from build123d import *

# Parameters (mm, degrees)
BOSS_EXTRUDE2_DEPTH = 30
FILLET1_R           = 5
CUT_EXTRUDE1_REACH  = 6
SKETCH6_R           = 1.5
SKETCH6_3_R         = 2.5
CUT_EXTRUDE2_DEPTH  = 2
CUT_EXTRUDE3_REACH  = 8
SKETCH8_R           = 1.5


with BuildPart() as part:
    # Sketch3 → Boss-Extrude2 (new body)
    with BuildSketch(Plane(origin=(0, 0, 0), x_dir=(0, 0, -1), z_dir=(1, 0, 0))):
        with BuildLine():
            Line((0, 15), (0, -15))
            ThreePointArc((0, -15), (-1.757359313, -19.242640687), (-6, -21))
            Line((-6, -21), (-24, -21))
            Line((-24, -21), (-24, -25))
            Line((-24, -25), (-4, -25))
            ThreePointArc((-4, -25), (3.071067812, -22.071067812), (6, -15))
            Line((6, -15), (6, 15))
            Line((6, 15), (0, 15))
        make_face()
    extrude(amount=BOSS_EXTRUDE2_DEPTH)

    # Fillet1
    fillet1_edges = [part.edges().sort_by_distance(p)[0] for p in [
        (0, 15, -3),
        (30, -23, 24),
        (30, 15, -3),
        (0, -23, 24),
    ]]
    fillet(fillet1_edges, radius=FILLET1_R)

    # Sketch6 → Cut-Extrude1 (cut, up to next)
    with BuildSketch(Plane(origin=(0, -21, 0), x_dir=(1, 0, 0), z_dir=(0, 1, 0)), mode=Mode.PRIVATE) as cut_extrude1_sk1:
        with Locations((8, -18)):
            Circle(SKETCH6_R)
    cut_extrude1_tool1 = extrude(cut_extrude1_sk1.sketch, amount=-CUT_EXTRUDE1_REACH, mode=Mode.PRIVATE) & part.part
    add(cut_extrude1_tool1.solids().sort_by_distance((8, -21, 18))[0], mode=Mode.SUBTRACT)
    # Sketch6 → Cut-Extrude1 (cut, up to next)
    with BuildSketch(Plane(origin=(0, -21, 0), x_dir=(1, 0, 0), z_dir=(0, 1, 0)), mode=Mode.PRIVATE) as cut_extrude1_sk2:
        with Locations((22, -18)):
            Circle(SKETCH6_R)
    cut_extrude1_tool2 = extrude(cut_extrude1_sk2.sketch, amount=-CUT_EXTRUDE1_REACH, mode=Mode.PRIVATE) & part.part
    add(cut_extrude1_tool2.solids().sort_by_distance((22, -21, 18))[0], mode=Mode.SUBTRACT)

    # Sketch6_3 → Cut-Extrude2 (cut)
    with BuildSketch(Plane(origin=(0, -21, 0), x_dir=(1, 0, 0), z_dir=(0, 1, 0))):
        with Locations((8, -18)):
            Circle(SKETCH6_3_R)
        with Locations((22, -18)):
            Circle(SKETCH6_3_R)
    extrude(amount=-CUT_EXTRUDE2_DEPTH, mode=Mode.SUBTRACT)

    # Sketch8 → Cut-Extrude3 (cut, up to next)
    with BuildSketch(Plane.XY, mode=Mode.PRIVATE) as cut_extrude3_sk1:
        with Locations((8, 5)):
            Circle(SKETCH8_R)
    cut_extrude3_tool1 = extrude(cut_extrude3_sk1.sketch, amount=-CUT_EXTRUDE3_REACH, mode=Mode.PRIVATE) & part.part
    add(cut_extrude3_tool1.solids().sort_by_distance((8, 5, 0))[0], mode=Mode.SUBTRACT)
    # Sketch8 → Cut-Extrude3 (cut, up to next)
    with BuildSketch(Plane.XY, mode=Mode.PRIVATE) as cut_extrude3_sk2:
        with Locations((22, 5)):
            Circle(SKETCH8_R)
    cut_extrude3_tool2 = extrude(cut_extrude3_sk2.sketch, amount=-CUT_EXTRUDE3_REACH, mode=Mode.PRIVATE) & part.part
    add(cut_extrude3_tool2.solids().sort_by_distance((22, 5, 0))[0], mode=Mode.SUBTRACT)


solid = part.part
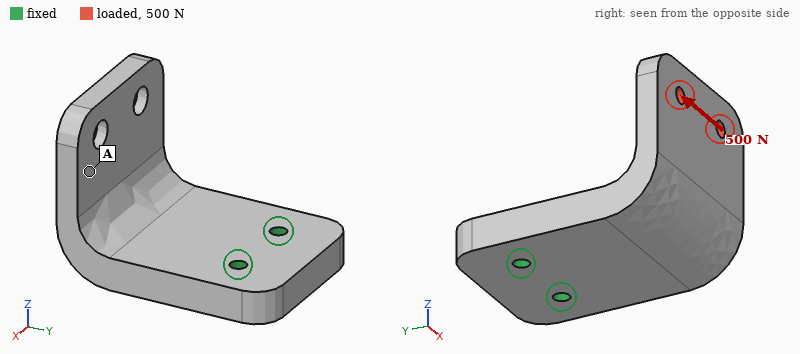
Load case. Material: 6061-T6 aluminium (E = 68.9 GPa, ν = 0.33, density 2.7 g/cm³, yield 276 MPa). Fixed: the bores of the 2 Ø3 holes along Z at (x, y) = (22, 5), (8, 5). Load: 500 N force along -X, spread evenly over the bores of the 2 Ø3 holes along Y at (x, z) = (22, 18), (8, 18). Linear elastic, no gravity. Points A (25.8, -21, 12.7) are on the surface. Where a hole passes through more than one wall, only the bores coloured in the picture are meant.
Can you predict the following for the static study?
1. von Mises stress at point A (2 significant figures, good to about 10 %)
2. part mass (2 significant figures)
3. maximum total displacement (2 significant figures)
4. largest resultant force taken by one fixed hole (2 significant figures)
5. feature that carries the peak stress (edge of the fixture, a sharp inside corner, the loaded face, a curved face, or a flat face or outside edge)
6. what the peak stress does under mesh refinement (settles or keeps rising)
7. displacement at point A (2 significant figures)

11 MPa
25 g
0.14 mm
1.1 kN
edge of the fixture
keeps rising
0.091 mm
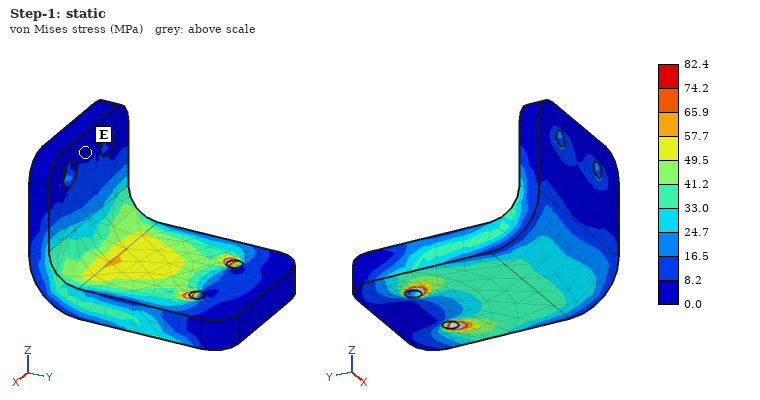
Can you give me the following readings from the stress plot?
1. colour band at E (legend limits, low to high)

0.0 to 8.2 MPa
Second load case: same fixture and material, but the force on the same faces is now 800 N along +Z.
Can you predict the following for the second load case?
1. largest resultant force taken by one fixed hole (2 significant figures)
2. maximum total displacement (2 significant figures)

400 N
0.34 mm
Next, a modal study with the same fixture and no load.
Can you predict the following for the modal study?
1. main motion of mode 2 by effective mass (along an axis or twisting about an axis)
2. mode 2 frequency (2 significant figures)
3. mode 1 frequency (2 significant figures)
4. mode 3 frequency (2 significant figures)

along X
4500 Hz
2600 Hz
6600 Hz
